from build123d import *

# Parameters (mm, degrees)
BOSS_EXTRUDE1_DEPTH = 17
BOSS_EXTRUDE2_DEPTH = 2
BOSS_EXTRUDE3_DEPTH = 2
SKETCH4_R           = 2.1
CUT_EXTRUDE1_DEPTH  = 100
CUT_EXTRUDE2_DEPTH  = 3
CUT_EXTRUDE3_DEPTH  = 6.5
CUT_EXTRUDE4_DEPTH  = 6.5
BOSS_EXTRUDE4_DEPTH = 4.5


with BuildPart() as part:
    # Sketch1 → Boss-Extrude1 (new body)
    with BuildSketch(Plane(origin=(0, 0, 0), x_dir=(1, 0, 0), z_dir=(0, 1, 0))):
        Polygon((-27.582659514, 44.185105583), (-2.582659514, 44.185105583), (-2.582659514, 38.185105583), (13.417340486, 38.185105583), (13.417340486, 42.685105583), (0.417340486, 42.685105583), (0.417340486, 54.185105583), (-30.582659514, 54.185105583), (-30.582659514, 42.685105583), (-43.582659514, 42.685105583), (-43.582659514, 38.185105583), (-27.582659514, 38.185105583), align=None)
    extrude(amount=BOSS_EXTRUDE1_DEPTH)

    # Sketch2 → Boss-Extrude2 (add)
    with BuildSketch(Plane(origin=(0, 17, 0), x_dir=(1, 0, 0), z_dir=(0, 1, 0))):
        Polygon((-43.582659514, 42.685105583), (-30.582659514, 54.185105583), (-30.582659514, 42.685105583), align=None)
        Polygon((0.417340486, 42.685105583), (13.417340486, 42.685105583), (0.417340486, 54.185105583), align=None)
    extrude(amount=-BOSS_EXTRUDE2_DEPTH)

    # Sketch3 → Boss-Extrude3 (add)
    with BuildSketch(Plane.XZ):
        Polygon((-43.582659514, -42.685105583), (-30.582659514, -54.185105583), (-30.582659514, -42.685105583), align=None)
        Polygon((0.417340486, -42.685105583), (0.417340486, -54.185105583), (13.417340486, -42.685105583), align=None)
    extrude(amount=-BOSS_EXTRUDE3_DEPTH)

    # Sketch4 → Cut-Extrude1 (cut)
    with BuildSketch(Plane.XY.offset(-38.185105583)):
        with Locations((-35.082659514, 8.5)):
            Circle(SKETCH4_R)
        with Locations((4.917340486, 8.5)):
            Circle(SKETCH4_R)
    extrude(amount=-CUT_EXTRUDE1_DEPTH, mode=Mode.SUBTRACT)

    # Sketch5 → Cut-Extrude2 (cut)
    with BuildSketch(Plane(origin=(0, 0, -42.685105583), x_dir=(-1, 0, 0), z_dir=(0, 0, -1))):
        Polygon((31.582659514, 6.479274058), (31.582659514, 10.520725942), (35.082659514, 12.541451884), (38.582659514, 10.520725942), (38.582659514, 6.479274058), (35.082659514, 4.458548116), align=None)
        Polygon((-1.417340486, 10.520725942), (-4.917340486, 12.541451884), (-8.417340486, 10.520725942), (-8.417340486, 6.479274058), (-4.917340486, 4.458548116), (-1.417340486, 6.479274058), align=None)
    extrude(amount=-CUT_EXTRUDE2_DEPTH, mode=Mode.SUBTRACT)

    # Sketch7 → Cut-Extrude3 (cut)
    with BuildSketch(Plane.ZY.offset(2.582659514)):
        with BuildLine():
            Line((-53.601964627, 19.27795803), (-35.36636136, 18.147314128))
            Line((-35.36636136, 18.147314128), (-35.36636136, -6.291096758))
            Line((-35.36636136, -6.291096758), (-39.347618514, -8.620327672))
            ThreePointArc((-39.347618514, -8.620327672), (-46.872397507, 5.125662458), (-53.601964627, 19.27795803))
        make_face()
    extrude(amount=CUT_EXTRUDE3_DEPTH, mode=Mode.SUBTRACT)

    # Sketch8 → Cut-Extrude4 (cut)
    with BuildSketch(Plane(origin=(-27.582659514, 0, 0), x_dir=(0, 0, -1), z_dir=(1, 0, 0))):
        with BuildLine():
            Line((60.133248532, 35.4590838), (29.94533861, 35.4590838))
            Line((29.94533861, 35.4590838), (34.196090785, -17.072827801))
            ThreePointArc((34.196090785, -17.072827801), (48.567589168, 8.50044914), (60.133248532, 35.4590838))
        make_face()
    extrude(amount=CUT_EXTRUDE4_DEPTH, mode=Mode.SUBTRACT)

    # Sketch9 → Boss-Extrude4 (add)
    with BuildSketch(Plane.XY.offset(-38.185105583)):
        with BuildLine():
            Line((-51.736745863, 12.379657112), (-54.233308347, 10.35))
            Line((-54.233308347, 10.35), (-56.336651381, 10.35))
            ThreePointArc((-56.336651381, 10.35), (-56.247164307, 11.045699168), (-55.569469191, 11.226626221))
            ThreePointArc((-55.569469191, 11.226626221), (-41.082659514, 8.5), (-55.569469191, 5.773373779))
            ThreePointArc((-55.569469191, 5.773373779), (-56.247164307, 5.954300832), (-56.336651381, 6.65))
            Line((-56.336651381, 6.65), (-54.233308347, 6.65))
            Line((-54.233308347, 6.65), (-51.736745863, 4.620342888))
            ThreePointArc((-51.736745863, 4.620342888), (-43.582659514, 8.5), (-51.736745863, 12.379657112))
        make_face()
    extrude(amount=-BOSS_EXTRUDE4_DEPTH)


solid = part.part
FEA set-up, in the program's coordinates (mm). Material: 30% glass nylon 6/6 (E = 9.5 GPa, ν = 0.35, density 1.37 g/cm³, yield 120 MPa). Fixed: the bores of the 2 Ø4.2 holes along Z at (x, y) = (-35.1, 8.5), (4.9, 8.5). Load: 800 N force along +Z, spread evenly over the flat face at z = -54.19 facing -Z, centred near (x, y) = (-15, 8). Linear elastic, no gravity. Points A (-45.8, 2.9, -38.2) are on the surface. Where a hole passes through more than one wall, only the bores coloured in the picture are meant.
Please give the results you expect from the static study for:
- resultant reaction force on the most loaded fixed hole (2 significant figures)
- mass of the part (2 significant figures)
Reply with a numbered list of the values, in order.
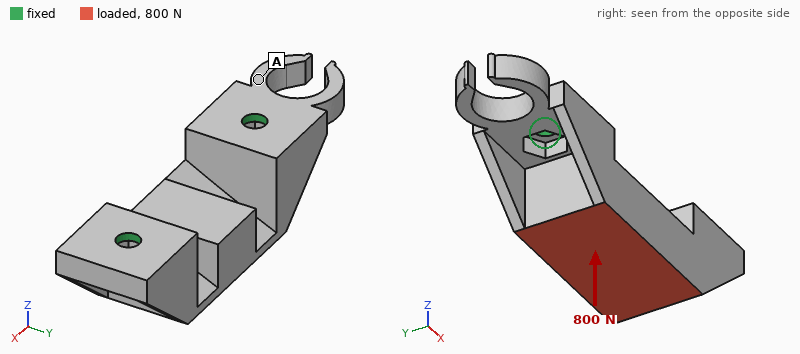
1. 470 N
2. 10 g
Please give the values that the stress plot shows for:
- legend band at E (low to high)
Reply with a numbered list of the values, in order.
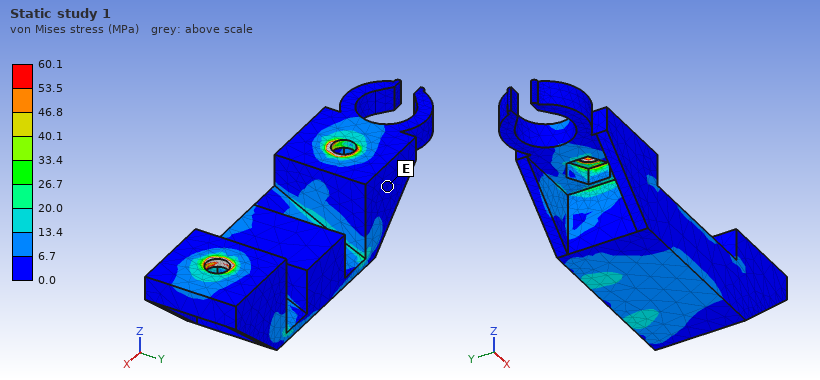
1. 0.0 to 6.7 MPa
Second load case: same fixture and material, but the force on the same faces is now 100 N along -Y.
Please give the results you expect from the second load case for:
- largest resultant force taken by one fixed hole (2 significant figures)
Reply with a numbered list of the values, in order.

1. 51 N
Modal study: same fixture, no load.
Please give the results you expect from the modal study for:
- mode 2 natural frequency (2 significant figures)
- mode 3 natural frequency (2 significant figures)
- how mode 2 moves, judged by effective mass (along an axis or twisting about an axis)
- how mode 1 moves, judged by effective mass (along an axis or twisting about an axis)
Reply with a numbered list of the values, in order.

1. 4500 Hz
2. 5100 Hz
3. along X
4. along Y
